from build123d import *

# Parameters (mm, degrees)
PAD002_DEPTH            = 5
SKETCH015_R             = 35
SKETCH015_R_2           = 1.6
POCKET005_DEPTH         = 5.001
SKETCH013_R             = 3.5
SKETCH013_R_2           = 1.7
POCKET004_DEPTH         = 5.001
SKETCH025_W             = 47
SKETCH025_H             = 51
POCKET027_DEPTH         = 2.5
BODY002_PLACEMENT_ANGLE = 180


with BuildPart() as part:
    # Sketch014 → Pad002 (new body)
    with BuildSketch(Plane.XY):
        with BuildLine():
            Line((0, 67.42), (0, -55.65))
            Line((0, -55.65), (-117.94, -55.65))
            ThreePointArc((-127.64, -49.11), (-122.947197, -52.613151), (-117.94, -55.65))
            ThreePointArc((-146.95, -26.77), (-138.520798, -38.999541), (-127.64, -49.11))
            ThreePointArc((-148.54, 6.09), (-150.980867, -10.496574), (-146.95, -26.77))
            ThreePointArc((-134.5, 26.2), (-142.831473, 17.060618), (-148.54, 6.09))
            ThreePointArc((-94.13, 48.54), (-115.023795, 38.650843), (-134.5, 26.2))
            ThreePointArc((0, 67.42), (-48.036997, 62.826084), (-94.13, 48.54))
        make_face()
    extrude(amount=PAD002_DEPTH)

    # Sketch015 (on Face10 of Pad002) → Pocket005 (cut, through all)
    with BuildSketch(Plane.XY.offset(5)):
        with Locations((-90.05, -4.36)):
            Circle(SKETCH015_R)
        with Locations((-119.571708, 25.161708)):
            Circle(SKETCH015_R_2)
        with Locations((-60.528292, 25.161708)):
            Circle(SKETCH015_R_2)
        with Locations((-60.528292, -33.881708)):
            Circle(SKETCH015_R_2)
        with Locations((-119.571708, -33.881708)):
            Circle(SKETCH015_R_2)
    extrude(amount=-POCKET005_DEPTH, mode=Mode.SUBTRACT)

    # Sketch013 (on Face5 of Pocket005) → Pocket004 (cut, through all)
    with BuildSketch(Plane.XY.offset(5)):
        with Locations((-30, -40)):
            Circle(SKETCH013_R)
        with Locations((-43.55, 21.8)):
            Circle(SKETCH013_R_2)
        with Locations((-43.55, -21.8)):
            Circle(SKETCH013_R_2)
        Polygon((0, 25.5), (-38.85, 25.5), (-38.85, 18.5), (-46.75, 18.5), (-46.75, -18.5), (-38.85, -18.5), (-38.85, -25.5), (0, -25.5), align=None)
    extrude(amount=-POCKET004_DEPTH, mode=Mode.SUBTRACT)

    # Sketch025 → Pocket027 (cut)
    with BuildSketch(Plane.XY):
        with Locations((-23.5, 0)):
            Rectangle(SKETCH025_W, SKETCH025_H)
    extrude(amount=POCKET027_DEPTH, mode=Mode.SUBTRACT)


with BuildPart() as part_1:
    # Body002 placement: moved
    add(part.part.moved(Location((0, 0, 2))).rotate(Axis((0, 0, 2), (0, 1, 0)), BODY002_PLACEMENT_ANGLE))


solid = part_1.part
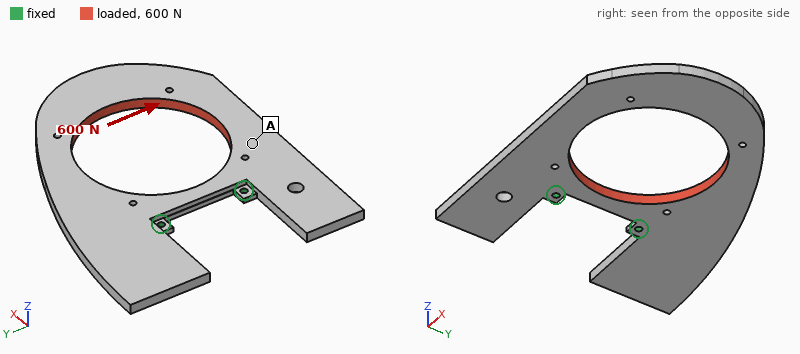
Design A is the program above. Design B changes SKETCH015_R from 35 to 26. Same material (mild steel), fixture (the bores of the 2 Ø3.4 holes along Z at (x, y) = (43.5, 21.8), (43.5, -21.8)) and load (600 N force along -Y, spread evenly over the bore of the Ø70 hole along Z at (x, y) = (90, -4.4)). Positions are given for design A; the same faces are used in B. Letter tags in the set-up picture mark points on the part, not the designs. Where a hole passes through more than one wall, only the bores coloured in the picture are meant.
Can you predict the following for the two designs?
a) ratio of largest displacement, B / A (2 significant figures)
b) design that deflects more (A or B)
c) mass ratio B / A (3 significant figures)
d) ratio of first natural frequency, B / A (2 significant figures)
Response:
0.35
A
1.19
0.98
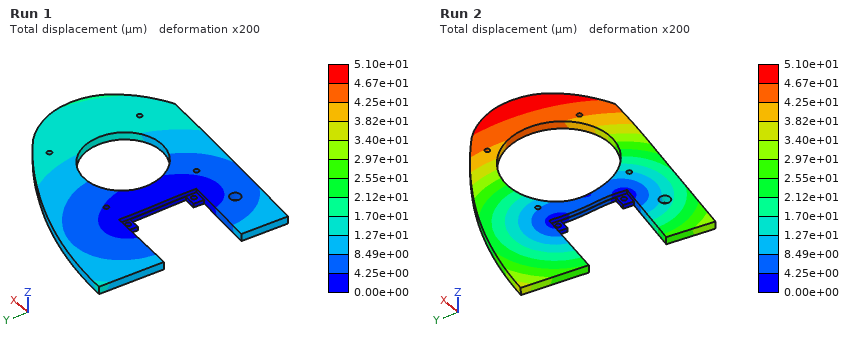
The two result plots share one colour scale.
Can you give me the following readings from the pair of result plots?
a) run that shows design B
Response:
Run 1
